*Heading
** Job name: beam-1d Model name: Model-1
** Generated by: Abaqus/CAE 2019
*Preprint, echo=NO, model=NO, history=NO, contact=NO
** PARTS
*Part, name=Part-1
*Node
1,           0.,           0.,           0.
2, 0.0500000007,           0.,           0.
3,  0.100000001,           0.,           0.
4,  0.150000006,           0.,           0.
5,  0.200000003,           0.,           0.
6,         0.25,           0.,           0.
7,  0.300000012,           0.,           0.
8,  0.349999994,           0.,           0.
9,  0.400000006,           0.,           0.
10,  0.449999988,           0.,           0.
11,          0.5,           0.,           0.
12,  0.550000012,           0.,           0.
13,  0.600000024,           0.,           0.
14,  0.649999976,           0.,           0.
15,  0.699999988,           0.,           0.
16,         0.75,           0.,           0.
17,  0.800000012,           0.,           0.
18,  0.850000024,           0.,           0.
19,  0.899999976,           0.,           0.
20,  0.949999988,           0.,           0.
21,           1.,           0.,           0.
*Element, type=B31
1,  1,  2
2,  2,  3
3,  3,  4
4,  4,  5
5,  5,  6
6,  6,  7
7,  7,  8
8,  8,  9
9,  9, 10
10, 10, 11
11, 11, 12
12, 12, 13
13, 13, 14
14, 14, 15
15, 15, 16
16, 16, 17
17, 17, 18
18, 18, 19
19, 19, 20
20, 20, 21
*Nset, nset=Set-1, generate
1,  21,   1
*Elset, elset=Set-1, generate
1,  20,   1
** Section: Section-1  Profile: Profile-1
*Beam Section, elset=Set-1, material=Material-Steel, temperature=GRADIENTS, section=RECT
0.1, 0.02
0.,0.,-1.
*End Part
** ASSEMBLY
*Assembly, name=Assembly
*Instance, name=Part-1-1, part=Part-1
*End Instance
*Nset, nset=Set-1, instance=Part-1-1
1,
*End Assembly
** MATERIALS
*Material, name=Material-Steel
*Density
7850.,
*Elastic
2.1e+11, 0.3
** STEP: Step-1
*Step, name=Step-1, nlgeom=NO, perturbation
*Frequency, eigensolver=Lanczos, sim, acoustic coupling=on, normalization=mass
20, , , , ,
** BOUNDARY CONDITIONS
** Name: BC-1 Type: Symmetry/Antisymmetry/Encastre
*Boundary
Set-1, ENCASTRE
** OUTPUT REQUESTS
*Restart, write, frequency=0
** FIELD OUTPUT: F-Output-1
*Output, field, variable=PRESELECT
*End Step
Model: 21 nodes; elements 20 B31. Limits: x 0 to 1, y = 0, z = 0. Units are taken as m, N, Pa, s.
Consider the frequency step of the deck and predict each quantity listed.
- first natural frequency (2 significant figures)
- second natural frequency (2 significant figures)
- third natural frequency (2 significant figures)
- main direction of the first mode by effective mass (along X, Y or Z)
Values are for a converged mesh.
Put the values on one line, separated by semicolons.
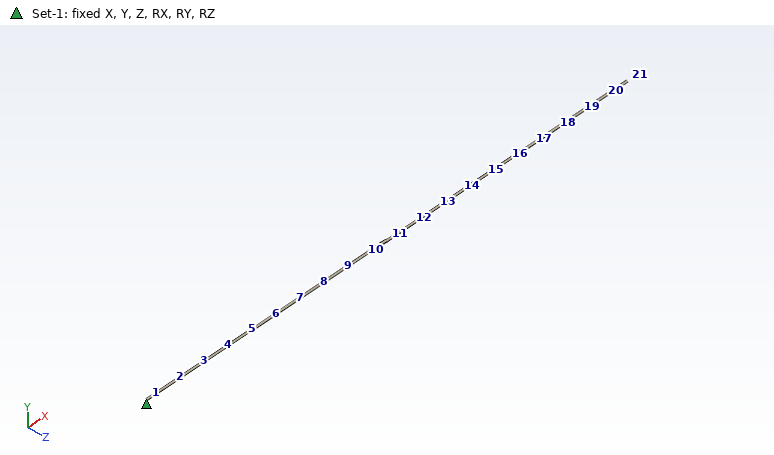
17 Hz; 83 Hz; 100 Hz; along Y
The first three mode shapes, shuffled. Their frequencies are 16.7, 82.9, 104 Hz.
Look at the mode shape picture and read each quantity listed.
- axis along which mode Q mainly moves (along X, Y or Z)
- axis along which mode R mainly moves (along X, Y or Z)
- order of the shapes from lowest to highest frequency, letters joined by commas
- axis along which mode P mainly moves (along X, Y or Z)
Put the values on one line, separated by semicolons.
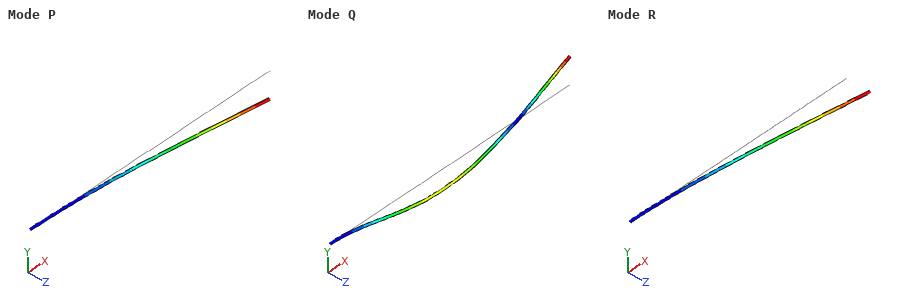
along Y; along Z; P, R, Q; along Y
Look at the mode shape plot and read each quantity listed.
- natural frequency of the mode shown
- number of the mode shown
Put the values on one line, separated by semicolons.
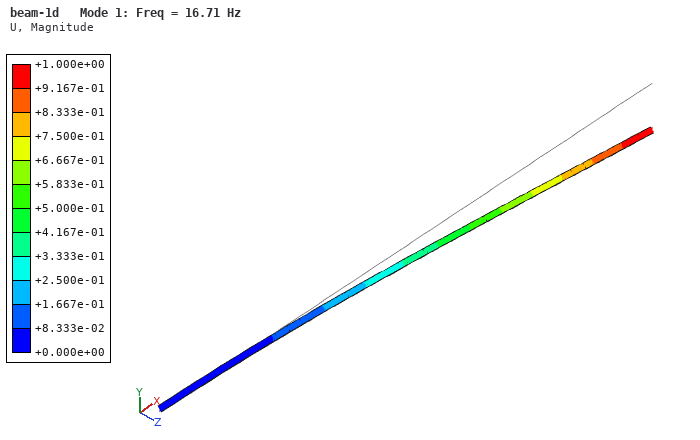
16.71 Hz; 1
